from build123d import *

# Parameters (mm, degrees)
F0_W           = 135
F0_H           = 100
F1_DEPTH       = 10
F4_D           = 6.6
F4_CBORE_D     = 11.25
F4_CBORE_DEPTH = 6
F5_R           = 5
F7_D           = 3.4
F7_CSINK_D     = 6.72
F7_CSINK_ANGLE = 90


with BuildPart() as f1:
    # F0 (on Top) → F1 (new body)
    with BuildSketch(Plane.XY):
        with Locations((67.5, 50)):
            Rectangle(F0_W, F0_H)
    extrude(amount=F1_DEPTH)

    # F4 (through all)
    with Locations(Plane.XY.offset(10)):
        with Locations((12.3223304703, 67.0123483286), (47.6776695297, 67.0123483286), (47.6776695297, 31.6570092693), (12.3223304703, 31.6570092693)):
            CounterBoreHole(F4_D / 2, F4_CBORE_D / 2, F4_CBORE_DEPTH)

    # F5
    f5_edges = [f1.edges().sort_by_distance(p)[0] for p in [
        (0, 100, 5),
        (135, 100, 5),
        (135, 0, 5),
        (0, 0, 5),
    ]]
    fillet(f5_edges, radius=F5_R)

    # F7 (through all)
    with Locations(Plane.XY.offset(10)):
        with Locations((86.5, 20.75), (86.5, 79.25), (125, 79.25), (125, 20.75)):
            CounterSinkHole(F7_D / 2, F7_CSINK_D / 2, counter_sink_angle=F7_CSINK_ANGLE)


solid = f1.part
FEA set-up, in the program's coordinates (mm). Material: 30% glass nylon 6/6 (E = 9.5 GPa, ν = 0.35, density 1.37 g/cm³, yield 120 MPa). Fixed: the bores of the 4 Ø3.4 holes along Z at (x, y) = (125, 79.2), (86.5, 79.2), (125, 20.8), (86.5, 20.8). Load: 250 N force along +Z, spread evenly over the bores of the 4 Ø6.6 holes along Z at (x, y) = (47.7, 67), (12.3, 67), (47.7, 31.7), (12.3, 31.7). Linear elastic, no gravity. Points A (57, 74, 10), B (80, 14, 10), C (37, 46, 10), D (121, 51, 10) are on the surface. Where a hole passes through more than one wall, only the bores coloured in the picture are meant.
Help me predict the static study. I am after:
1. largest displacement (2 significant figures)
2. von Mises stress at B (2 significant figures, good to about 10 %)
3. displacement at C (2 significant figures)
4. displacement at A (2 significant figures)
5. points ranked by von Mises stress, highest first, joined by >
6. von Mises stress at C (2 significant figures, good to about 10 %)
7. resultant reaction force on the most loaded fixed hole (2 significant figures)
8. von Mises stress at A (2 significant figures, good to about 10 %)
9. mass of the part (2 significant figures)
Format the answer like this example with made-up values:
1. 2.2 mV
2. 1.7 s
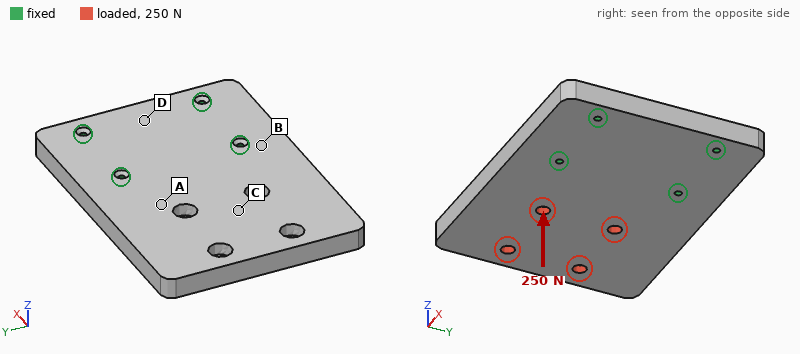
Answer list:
1. 0.49 mm
2. 7.1 MPa
3. 0.23 mm
4. 0.11 mm
5. B > A > C > D
6. 2.4 MPa
7. 250 N
8. 4.0 MPa
9. 180 g
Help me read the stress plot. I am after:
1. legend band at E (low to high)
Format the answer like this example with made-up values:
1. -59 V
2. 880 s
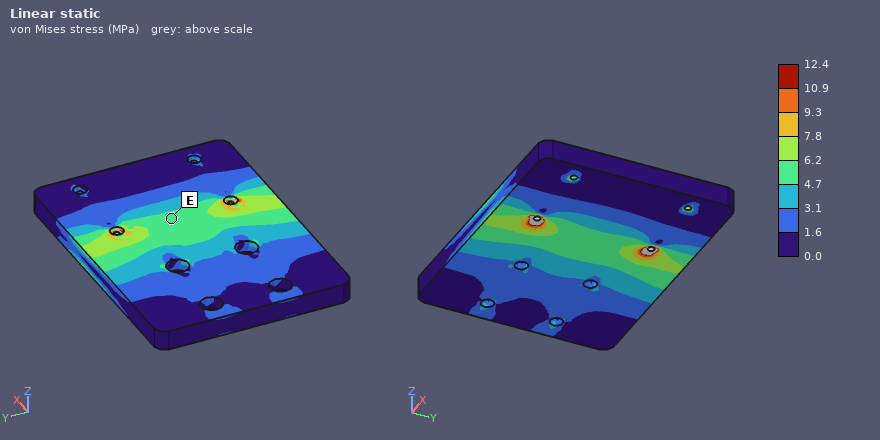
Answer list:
1. 4.7 to 6.2 MPa
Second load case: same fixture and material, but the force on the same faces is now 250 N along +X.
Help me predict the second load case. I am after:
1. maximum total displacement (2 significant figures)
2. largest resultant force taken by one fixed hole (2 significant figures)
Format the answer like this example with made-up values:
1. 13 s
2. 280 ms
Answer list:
1. 35 µm
2. 96 N
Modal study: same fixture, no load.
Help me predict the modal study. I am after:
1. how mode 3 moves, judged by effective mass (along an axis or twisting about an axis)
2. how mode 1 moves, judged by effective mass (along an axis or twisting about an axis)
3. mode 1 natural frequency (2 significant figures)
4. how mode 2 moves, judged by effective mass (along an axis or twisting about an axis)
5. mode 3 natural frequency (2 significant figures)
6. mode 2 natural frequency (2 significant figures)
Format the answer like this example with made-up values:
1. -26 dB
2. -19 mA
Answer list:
1. along Y
2. along Z
3. 510 Hz
4. twisting about X
5. 2700 Hz
6. 1100 Hz
